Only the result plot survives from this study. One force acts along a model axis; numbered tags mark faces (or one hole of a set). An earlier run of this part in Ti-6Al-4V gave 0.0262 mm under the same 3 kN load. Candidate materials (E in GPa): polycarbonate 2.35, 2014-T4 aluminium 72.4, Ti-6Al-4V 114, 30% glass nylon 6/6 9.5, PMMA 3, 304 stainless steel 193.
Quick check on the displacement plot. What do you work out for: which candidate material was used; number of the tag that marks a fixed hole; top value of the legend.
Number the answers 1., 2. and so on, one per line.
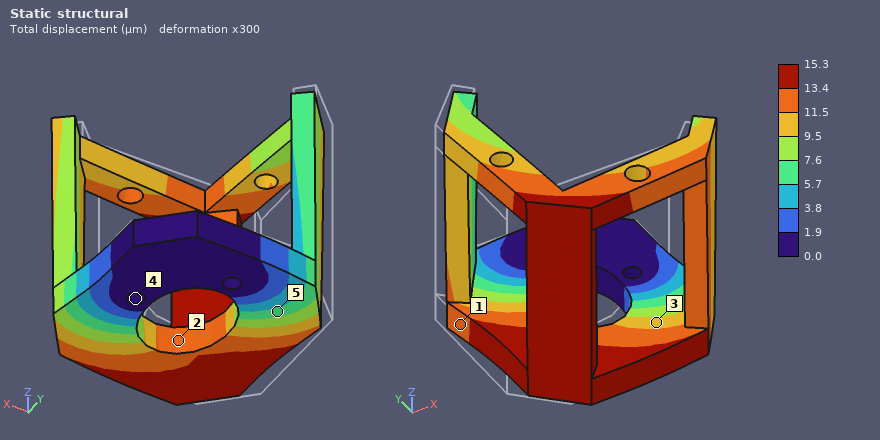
1. 304 stainless steel
2. 4
3. 15.3 µm
